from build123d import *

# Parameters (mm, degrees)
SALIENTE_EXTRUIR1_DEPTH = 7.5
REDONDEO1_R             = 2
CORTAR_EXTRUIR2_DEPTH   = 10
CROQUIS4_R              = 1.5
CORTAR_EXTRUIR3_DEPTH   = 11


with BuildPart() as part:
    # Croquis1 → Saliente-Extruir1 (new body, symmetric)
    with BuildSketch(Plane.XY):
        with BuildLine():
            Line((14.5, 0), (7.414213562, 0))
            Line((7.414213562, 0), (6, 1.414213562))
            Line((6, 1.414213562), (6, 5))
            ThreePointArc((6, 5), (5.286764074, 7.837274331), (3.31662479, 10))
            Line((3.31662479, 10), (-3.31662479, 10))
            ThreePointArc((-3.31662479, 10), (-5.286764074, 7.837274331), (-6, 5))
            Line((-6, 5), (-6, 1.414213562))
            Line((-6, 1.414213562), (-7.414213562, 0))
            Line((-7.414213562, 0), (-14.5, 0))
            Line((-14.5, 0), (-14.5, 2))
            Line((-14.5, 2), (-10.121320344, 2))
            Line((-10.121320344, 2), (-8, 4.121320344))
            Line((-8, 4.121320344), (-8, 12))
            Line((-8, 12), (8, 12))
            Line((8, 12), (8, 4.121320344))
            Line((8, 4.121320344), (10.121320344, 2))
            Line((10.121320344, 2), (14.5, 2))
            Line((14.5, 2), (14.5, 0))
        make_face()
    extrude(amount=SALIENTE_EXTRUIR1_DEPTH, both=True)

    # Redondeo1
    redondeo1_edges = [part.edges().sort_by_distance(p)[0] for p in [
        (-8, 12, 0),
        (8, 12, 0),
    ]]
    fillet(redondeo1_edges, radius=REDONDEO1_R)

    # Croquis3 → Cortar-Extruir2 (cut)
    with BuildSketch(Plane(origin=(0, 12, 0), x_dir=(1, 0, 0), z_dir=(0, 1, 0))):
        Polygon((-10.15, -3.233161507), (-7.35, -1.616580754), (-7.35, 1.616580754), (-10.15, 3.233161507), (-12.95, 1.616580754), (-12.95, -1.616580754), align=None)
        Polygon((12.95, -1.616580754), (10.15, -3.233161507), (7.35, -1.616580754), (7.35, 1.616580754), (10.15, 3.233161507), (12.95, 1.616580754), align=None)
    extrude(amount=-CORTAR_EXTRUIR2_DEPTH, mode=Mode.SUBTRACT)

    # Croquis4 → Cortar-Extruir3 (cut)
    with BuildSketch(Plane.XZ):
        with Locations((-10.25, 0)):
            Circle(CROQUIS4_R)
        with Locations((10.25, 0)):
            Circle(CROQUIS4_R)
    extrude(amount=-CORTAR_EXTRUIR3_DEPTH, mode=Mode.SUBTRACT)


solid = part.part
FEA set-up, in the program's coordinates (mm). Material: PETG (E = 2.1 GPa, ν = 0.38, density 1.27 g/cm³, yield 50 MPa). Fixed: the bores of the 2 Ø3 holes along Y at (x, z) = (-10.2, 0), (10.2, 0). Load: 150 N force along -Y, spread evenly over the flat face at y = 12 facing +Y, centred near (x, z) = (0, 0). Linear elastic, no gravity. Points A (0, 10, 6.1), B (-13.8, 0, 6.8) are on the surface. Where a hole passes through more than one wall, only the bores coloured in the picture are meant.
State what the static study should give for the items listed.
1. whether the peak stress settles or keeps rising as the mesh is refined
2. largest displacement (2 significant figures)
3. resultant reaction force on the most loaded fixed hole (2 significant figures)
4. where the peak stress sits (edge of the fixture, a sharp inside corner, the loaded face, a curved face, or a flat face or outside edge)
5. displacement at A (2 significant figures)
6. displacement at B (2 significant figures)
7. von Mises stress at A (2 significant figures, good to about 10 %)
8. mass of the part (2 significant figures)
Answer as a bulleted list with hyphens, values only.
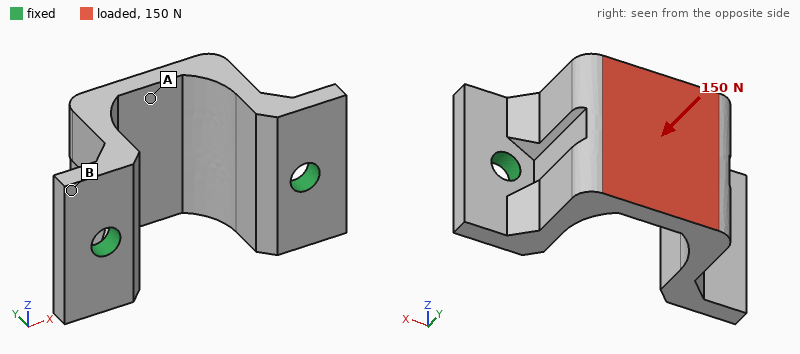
- keeps rising
- 75 µm
- 83 N
- edge of the fixture
- 71 µm
- 21 µm
- 5.4 MPa
- 1.9 g
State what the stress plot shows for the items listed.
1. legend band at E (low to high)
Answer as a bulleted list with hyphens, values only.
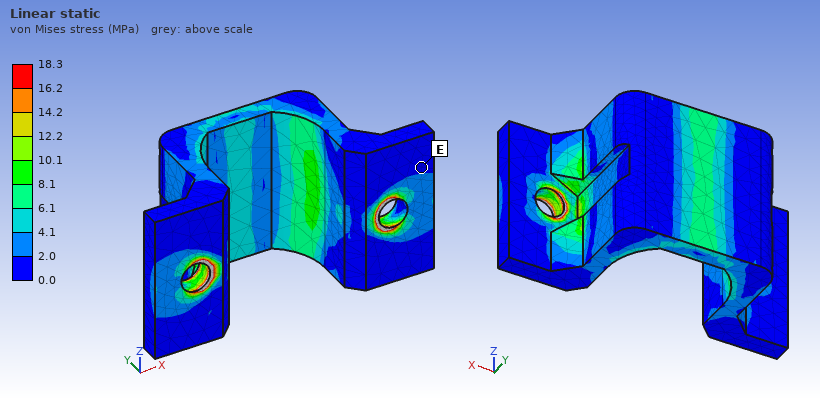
- 0.0 to 2.0 MPa
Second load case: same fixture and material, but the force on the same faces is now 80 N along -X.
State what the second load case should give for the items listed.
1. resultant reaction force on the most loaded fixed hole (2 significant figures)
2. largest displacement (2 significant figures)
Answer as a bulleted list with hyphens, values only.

- 56 N
- 0.12 mm
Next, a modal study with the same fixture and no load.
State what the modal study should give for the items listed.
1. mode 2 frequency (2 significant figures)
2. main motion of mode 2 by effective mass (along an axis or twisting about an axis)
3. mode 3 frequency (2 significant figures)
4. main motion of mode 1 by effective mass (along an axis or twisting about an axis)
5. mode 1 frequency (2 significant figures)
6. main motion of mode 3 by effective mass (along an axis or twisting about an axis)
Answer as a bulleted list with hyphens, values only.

- 4200 Hz
- along X
- 4500 Hz
- along Z
- 2500 Hz
- twisting about Y
